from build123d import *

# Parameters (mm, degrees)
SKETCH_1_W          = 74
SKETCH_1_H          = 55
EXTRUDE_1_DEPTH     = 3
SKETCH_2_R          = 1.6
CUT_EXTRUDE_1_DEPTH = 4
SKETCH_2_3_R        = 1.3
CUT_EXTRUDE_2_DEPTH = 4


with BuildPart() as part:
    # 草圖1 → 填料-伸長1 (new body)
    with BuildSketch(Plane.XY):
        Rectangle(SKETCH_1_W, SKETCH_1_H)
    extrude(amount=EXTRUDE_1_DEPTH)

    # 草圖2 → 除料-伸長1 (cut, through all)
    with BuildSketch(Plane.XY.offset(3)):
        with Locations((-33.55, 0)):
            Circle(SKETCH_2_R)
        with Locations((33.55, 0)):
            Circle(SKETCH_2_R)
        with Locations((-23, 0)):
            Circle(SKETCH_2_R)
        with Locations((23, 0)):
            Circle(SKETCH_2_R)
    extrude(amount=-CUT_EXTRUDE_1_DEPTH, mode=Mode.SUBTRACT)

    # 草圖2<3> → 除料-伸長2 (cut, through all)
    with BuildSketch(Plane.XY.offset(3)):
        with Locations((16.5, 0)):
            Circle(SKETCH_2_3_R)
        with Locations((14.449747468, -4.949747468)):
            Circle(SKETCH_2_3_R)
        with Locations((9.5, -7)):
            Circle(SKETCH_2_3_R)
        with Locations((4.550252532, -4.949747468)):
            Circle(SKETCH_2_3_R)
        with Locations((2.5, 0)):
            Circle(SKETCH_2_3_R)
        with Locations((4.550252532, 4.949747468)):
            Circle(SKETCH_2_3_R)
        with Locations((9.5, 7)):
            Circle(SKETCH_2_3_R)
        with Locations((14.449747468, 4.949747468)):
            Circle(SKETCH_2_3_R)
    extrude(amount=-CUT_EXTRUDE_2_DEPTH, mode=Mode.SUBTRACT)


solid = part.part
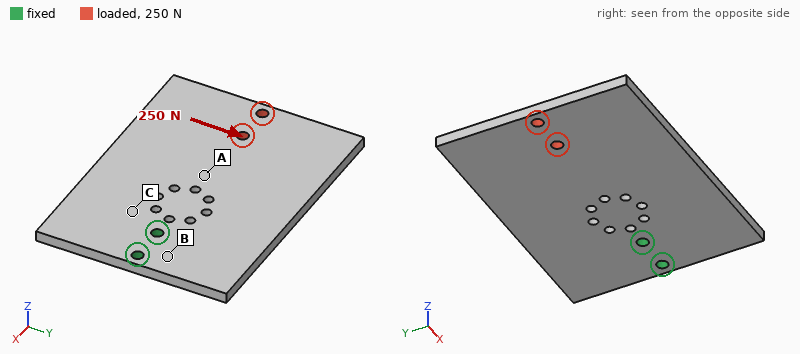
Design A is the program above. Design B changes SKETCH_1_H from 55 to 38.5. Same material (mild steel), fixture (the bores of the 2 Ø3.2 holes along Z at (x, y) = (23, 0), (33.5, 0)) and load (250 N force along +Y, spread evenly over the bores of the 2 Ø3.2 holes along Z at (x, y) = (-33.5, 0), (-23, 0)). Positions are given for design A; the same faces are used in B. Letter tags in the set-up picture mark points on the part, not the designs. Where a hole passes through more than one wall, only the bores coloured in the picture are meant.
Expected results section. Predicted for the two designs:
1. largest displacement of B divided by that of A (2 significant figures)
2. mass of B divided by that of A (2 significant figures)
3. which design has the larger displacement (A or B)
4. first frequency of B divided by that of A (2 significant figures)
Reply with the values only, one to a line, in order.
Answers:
1.2
0.69
B
1.1
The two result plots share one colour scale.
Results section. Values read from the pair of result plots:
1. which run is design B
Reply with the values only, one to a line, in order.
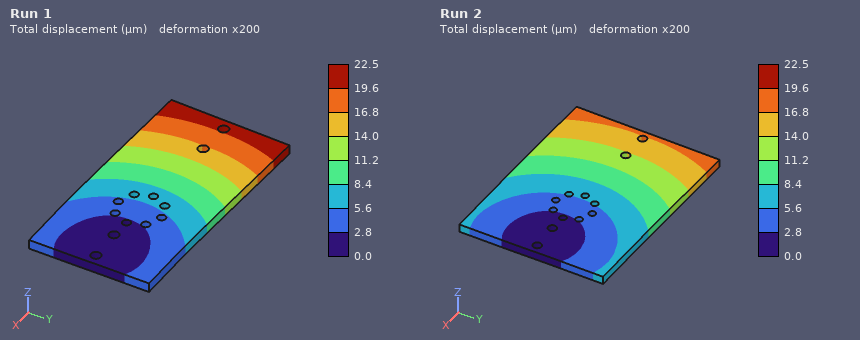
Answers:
Run 1
